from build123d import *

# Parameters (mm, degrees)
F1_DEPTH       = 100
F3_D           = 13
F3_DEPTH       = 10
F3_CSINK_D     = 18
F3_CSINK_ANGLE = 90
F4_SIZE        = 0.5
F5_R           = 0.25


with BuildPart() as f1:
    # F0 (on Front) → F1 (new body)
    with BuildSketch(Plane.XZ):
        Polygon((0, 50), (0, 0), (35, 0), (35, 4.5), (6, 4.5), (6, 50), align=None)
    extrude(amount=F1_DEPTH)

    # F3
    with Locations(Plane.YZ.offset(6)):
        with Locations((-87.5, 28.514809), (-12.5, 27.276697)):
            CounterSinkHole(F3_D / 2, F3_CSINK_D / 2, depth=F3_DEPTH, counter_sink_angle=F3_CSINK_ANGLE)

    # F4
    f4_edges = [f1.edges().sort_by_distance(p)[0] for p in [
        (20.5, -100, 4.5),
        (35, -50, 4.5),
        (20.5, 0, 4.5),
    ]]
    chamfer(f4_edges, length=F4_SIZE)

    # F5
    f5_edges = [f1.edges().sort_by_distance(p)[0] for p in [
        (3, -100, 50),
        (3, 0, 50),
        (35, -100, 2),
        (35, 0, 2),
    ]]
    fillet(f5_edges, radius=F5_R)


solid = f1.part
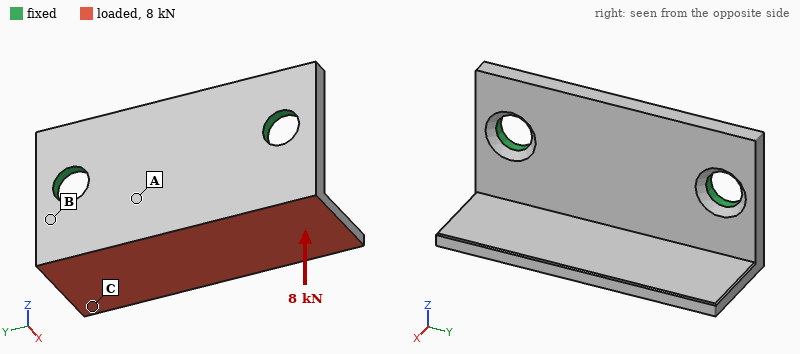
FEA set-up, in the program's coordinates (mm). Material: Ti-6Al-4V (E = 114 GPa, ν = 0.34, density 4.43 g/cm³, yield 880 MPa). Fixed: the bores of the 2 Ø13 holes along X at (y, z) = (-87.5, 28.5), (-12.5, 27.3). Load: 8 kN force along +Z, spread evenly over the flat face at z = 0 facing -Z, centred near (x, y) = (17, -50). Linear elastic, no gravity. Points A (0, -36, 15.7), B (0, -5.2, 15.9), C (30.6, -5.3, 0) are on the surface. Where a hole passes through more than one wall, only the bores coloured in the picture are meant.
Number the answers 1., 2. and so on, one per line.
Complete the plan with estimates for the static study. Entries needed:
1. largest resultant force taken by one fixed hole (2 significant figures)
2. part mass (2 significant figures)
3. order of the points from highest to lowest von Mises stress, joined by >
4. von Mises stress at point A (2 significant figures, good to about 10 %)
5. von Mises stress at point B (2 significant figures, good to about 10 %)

1. 4.1 kN
2. 180 g
3. B > A > C
4. 130 MPa
5. 220 MPa
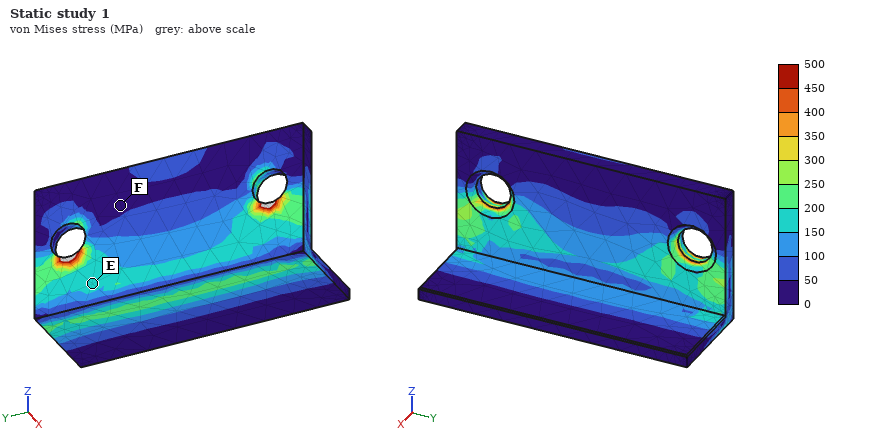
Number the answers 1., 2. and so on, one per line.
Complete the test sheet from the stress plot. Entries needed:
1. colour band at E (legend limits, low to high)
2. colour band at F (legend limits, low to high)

1. 150 to 200 MPa
2. 0 to 50 MPa
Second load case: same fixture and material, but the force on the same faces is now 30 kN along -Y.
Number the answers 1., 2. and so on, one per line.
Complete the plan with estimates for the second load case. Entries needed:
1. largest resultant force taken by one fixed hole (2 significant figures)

1. 19 kN
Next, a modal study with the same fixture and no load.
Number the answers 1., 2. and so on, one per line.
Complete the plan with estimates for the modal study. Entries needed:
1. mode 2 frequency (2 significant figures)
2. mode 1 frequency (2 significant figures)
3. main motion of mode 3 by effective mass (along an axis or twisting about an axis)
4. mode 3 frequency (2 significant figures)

1. 3100 Hz
2. 2100 Hz
3. along X
4. 4700 Hz
